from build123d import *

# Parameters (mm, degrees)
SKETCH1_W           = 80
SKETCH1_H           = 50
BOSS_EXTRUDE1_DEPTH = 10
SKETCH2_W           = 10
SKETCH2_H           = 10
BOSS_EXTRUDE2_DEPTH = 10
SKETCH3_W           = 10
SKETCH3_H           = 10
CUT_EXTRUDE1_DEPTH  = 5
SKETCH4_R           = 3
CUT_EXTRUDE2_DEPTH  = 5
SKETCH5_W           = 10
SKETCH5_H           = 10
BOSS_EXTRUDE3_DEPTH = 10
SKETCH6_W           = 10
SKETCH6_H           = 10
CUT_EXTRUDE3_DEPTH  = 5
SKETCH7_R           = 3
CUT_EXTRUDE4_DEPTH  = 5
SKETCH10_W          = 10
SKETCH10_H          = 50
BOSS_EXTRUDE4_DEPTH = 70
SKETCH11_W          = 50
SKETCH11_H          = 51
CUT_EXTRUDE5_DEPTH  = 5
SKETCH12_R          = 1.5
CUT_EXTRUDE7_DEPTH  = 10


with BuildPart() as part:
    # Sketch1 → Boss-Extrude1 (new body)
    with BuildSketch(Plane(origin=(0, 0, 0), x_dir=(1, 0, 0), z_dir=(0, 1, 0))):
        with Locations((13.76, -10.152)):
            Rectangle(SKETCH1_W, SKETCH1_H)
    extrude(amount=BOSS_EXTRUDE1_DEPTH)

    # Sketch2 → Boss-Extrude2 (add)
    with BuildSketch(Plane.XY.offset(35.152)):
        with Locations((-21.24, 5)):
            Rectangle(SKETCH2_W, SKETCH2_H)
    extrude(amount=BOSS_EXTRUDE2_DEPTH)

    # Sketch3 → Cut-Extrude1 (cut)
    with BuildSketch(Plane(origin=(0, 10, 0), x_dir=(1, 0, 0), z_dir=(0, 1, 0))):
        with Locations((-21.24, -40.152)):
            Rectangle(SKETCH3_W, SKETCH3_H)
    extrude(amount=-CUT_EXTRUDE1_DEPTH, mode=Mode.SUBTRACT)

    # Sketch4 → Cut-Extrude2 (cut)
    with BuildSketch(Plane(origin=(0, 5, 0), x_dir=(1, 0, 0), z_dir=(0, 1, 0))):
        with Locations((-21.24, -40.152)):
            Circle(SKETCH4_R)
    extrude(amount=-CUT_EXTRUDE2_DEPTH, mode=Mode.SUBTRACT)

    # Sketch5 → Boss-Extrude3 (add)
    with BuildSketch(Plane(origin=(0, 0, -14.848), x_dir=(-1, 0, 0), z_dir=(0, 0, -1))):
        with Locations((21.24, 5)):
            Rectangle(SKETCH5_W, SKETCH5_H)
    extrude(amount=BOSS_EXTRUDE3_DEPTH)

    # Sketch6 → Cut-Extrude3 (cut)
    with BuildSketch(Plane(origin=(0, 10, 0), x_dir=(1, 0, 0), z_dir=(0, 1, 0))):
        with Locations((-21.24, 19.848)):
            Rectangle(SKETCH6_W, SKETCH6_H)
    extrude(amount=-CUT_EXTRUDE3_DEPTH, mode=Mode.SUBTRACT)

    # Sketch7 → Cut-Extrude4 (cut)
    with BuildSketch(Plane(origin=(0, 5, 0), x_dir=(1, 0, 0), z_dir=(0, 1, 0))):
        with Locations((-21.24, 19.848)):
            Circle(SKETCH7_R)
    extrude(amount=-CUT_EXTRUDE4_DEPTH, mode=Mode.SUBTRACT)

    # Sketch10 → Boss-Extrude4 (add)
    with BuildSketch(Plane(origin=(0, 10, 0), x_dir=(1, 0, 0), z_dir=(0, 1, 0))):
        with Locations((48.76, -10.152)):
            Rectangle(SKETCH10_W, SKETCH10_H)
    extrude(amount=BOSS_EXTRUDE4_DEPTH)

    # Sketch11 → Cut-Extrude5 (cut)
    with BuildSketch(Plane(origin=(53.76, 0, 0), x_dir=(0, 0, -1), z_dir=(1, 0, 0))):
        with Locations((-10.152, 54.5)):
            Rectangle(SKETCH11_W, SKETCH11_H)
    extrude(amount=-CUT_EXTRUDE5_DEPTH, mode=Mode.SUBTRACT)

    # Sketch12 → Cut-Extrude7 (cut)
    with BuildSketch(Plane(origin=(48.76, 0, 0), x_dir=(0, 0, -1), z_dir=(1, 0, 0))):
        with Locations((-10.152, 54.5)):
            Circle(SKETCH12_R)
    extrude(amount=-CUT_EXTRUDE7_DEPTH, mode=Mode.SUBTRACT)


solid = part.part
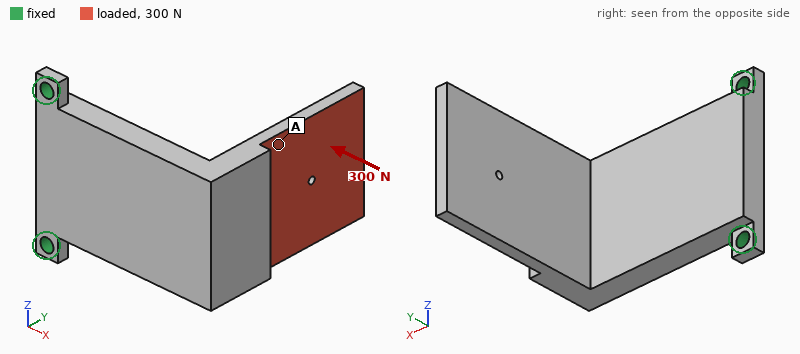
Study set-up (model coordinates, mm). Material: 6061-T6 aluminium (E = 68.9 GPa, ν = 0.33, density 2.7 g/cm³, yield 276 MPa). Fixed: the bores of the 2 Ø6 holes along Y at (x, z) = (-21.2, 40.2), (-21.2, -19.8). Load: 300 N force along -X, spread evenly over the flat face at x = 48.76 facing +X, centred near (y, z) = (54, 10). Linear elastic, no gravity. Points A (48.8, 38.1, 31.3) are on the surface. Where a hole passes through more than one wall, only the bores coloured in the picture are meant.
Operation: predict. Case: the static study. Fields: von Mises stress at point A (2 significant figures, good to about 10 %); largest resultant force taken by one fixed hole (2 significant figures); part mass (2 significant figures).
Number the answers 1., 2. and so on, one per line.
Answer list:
1. 24 MPa
2. 150 N
3. 170 g
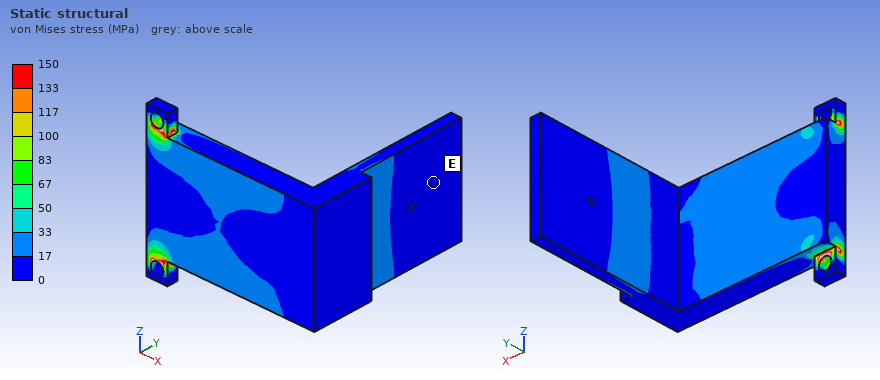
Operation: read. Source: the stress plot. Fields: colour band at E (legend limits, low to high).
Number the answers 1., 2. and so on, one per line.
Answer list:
1. 0 to 17 MPa
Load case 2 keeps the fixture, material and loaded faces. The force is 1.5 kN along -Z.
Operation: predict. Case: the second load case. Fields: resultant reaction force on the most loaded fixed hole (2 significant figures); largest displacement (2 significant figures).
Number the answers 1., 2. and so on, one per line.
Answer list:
1. 2.6 kN
2. 0.97 mm
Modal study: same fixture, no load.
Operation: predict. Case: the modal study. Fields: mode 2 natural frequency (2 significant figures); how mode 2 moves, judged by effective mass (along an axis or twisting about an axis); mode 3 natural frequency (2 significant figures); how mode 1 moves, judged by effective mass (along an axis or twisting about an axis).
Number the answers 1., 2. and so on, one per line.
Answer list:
1. 1100 Hz
2. along Z
3. 1200 Hz
4. along Y
